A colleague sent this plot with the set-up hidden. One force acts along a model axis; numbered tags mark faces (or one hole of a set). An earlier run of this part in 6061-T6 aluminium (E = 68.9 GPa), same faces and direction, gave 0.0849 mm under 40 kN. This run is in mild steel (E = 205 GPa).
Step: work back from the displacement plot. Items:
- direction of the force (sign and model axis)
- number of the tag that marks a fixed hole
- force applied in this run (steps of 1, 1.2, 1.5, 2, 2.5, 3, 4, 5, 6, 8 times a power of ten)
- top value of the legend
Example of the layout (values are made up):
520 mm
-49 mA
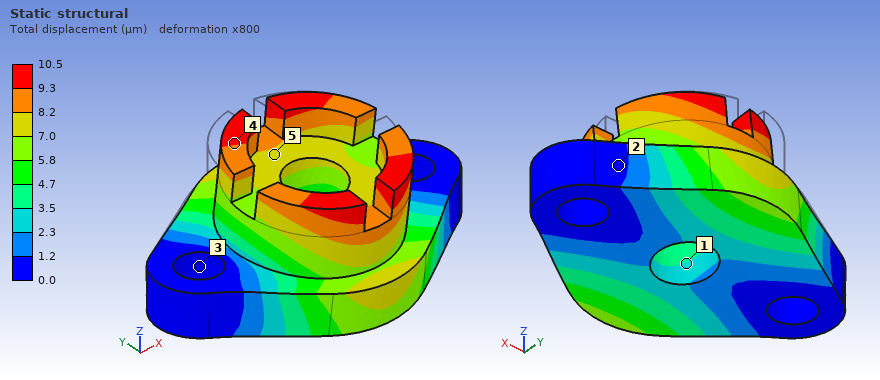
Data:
-Y
3
15 kN
10.5 µm
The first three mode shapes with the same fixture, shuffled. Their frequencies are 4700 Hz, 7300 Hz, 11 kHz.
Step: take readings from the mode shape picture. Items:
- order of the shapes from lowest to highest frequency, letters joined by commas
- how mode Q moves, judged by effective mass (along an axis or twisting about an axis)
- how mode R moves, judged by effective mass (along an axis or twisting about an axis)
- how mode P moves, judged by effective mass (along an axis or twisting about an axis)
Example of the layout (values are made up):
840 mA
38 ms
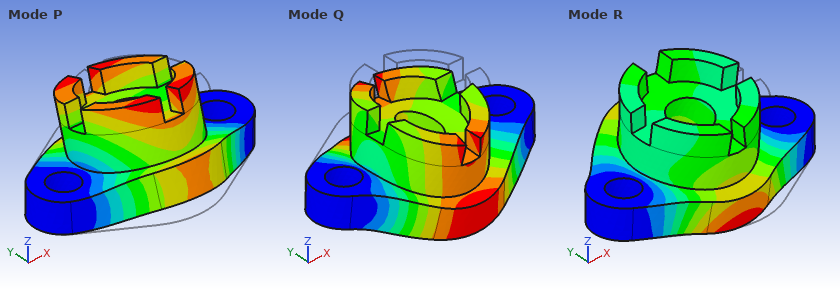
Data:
P, Q, R
along Z
along Y
along Y
